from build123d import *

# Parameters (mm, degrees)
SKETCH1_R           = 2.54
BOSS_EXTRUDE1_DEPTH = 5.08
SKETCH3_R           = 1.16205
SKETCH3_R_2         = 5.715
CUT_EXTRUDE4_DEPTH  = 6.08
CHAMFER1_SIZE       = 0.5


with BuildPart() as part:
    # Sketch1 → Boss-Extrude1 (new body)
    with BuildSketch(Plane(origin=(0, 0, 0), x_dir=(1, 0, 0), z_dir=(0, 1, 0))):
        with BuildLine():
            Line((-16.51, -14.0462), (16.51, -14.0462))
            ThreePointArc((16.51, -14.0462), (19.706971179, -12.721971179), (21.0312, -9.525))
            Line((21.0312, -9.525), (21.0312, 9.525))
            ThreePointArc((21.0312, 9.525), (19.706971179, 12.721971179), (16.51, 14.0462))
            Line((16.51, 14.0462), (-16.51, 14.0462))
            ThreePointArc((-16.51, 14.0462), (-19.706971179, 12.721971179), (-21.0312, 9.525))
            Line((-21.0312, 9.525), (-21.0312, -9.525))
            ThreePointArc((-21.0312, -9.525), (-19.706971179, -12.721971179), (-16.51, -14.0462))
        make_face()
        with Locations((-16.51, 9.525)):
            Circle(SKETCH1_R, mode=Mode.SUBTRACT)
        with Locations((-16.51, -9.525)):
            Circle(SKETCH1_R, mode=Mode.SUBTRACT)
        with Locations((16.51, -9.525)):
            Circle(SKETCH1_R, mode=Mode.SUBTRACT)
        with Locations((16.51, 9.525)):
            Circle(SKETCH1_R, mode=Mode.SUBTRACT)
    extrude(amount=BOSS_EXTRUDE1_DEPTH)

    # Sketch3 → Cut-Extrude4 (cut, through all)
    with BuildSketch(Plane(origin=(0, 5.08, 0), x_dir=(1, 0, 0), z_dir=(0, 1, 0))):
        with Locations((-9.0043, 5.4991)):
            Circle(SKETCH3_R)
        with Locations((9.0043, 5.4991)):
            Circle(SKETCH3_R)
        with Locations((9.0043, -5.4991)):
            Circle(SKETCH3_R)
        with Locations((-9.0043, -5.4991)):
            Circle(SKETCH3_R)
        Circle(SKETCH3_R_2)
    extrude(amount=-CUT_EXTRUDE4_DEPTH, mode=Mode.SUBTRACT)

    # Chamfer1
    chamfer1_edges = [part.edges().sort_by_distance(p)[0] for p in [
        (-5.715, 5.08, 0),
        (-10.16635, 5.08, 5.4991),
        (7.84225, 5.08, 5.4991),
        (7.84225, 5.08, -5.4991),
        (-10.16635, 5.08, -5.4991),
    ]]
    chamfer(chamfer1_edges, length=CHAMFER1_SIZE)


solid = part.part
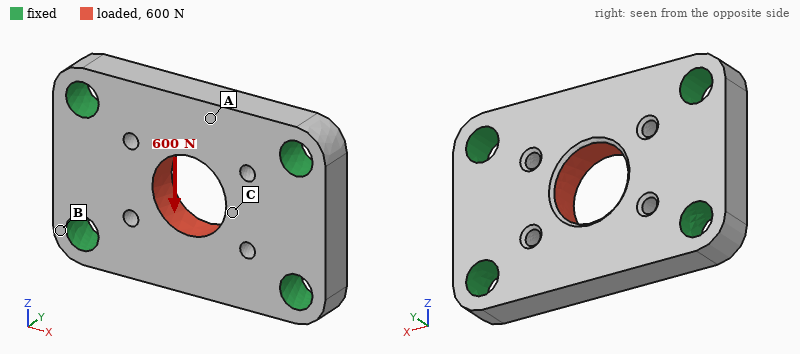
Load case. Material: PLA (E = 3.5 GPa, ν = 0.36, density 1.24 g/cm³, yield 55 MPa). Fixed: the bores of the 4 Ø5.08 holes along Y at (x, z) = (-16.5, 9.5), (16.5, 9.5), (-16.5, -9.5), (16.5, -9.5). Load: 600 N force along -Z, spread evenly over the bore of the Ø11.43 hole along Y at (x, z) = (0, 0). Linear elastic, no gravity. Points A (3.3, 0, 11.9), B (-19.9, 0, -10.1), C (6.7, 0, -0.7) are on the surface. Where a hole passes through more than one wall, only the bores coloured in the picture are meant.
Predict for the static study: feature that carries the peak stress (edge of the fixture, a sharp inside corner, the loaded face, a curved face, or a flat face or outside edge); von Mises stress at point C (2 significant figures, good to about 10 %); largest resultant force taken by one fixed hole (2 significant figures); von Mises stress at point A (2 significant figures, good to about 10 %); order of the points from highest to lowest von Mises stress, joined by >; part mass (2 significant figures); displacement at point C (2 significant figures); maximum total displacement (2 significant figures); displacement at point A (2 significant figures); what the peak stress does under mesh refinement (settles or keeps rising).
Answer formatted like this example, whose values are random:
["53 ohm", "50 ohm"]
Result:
["a sharp inside corner", "6.6 MPa", "180 N", "2.5 MPa", "C > A > B", "6.1 g", "21 µm", "33 µm", "26 µm", "keeps rising"]
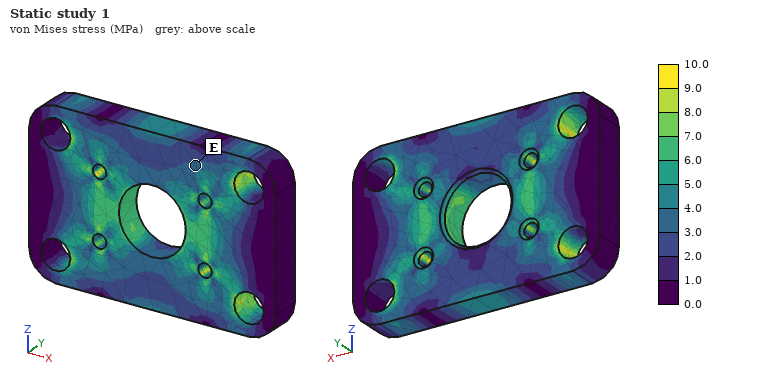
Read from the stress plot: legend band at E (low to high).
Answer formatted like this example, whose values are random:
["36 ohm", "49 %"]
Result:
["3.0 to 4.0 MPa"]
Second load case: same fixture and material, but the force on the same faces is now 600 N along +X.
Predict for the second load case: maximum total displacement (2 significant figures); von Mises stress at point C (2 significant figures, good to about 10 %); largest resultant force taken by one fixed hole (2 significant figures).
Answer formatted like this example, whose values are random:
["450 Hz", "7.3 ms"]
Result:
["14 µm", "3.7 MPa", "160 N"]
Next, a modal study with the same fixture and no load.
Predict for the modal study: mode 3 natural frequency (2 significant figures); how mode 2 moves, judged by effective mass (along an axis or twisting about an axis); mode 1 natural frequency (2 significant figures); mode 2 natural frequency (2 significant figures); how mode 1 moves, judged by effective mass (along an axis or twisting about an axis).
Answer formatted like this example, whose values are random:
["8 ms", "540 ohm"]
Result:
["14 kHz", "twisting about X", "8300 Hz", "9600 Hz", "along Y"]
